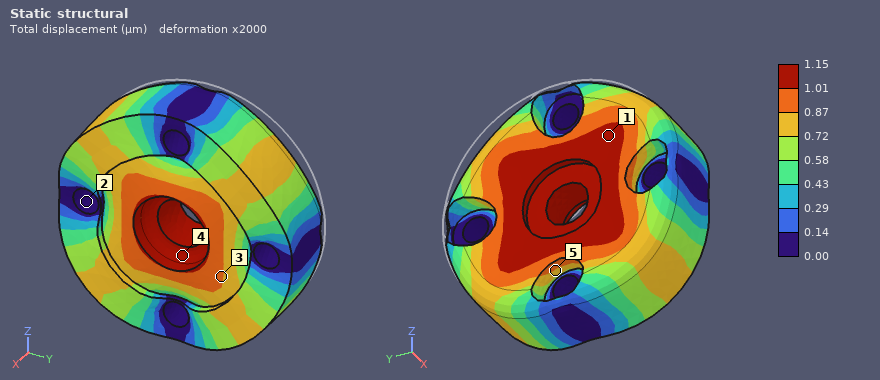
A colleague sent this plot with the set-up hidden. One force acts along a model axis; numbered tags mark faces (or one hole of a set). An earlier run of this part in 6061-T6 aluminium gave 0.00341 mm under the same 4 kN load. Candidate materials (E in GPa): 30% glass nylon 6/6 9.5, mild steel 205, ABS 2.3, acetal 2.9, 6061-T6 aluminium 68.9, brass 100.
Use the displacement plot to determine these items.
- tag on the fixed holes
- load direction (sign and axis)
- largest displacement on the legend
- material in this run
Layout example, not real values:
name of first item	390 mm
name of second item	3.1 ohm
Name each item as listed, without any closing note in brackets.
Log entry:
tag on the fixed holes	2
load direction	+X
largest displacement on the legend	1.15 µm
material in this run	mild steel
